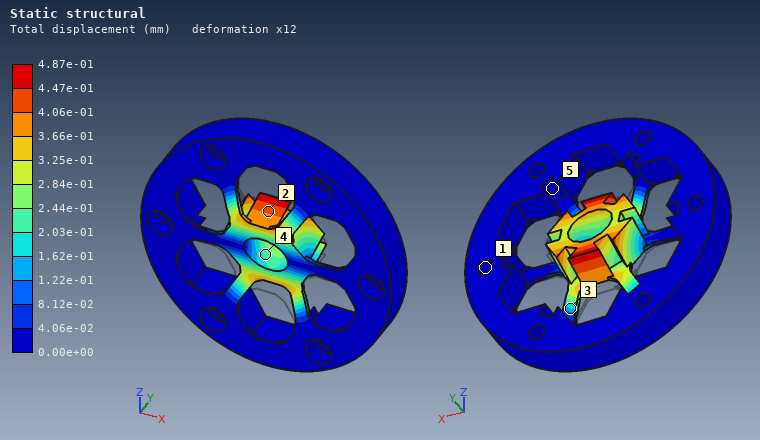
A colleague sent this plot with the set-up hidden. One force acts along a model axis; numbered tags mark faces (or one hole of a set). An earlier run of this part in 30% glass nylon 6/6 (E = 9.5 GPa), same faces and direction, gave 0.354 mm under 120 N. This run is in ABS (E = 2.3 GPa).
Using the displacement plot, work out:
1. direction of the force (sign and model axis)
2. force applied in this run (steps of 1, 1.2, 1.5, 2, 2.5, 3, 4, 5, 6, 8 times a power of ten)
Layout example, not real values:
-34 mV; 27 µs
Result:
+Z; 40 N
